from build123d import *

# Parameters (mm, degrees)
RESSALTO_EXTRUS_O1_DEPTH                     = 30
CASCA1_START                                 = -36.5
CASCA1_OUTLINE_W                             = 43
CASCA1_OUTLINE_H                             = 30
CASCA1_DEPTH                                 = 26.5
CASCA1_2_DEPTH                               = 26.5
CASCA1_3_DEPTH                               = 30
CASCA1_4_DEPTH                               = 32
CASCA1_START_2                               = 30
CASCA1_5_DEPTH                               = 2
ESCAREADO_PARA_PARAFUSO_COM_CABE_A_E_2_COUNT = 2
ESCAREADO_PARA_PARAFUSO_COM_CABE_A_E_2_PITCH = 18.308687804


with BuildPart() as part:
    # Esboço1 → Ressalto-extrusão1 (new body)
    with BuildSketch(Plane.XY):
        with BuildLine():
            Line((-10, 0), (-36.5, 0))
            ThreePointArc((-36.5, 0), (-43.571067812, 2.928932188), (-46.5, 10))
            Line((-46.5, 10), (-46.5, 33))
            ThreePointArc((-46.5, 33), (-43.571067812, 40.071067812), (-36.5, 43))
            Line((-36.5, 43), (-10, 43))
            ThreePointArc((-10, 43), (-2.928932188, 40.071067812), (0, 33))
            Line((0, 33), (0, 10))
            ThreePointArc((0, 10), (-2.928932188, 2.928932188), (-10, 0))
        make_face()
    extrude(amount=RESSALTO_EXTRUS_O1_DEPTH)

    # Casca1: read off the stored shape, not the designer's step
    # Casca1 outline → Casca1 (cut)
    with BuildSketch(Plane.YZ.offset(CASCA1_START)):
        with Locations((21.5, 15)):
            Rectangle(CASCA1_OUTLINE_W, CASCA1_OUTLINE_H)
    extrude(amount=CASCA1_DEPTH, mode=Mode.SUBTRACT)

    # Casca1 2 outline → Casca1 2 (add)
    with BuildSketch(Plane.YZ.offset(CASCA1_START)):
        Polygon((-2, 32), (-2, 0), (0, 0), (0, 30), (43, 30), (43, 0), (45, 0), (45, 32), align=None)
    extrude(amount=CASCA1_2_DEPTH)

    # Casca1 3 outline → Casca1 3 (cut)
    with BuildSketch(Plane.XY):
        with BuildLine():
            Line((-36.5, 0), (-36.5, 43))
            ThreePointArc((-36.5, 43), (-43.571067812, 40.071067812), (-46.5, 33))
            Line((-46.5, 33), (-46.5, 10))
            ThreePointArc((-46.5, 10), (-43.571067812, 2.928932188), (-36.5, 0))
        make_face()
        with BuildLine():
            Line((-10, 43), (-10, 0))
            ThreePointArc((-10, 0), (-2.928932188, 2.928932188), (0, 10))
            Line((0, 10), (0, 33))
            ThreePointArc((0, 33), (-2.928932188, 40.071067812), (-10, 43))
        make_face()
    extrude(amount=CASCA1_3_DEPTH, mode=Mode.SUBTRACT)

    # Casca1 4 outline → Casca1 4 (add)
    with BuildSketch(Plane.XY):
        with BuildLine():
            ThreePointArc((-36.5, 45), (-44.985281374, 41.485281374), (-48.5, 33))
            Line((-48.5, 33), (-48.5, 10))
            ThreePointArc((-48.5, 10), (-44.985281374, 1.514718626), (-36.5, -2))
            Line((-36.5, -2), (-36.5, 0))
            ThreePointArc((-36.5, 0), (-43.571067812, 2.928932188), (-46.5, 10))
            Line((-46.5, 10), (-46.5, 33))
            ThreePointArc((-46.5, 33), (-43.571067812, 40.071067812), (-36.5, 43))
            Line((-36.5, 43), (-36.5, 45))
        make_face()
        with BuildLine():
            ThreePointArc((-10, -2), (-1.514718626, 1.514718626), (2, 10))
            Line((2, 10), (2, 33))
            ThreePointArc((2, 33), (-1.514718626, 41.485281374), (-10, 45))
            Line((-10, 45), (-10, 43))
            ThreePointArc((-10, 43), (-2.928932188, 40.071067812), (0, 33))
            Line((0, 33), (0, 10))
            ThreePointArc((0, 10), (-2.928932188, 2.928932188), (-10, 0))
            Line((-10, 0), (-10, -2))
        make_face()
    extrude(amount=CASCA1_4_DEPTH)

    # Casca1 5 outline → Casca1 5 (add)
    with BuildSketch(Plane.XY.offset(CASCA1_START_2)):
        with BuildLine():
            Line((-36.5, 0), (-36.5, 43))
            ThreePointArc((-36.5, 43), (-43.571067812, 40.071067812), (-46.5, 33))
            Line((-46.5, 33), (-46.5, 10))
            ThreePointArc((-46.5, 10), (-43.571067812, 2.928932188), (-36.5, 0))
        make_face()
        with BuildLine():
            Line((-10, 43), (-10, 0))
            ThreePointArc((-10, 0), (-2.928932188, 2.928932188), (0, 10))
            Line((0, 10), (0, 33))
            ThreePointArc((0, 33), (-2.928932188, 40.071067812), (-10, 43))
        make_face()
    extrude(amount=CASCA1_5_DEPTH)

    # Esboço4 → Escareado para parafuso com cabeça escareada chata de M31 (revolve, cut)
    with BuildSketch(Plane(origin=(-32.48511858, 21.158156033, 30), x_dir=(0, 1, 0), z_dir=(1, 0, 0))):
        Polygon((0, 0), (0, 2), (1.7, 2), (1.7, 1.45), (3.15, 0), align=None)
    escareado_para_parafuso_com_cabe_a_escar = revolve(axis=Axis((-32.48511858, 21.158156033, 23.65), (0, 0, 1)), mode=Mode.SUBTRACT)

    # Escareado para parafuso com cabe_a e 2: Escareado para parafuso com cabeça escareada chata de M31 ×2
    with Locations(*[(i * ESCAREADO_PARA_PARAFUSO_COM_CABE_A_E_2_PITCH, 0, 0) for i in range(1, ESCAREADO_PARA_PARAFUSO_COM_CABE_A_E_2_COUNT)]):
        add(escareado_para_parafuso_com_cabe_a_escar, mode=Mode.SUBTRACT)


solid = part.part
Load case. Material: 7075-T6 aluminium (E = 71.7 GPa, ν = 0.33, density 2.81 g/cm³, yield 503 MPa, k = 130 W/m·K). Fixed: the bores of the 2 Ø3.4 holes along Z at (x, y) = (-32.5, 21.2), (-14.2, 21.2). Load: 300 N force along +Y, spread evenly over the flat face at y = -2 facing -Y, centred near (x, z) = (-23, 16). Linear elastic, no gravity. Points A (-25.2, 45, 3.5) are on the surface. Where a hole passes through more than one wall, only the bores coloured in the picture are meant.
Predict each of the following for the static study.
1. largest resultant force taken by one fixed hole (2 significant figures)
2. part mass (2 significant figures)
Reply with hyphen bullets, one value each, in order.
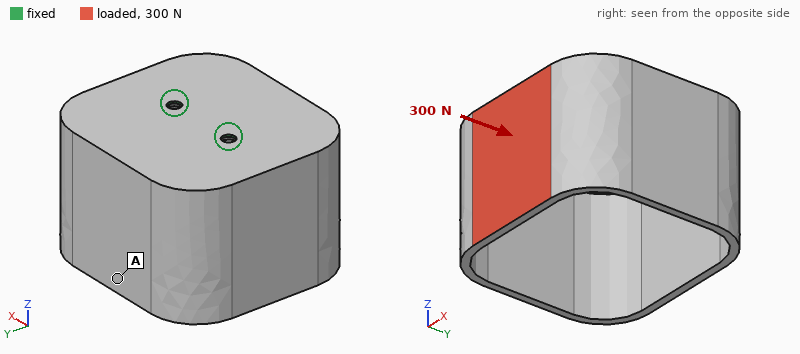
- 160 N
- 41 g
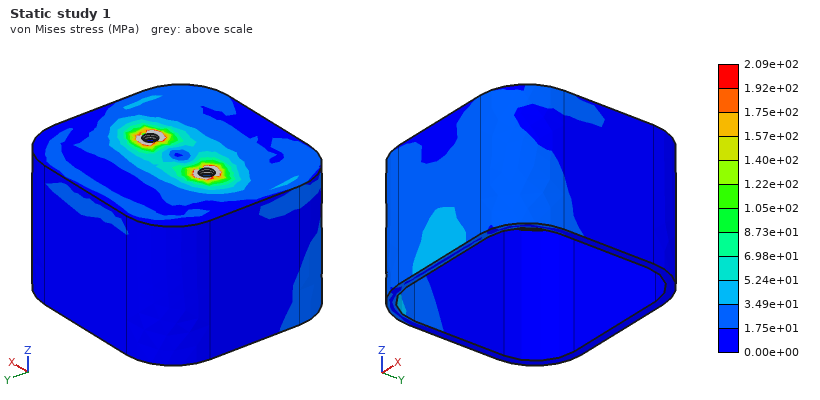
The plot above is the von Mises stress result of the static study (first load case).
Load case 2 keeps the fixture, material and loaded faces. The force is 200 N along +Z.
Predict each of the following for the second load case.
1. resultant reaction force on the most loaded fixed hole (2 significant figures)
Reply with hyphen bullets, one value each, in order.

- 150 N
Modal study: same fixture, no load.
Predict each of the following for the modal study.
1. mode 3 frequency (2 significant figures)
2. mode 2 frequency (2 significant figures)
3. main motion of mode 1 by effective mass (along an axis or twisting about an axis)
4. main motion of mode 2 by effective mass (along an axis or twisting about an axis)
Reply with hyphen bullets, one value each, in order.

- 2000 Hz
- 1200 Hz
- along Y
- along X
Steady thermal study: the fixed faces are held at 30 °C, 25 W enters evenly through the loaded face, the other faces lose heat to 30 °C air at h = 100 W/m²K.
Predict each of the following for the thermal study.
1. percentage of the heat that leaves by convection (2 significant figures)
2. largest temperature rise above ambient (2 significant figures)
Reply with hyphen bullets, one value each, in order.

- 63 %
- 36 K
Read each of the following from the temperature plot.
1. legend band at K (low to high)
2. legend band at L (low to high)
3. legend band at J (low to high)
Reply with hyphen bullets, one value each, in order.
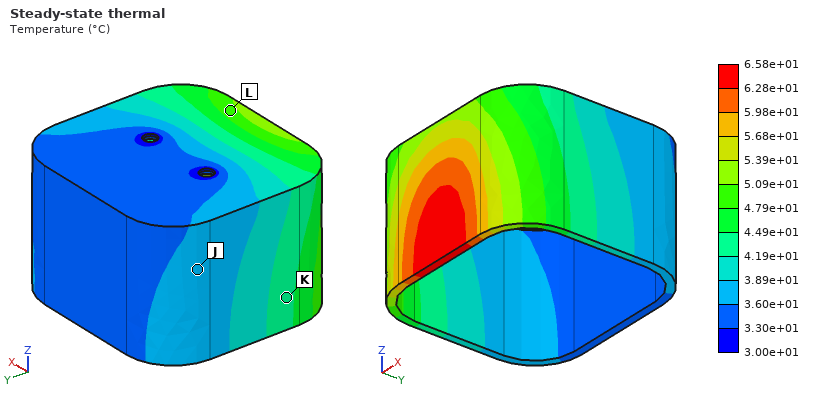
- 4.19e+01 to 4.49e+01 °C
- 4.79e+01 to 5.09e+01 °C
- 3.60e+01 to 3.89e+01 °C
